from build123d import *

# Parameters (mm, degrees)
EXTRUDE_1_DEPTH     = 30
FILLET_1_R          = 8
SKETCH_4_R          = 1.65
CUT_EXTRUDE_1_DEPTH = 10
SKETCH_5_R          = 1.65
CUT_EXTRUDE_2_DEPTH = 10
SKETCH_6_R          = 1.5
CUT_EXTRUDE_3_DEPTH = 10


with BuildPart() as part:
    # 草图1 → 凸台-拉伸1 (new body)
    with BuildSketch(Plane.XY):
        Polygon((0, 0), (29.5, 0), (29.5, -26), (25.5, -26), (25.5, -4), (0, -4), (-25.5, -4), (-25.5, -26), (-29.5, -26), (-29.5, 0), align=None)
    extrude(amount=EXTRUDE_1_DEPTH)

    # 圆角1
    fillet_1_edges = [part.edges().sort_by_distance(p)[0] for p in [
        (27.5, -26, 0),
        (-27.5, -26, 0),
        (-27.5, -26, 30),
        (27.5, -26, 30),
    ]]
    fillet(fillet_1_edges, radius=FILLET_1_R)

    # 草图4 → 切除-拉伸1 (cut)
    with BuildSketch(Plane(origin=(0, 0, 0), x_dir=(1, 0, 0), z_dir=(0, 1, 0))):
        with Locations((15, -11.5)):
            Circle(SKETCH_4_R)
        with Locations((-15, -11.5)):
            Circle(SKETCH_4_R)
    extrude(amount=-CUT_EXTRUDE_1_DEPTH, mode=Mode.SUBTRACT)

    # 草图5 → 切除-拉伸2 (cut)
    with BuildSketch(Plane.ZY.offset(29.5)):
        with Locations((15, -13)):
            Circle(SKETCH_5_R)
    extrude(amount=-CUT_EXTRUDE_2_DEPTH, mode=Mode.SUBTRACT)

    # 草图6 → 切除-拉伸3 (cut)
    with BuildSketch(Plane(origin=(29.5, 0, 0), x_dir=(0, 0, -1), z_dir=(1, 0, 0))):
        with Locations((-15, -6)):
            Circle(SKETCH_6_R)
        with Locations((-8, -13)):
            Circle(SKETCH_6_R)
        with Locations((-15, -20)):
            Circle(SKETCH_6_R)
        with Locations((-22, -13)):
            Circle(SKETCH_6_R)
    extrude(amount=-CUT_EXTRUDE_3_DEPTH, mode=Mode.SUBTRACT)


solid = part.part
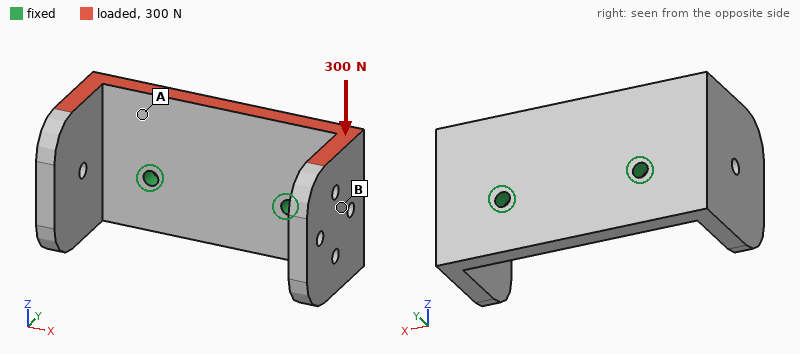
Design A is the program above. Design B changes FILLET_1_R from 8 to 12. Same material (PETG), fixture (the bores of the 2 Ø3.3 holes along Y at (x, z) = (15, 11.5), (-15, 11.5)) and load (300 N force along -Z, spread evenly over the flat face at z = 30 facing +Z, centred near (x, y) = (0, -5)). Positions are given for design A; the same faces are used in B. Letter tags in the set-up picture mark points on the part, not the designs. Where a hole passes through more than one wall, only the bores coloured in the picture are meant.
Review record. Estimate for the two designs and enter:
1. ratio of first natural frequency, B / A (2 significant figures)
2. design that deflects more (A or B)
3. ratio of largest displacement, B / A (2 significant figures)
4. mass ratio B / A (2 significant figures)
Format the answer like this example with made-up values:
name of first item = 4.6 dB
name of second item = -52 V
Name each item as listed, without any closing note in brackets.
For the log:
ratio of first natural frequency, B / A = 1.1
design that deflects more = A
ratio of largest displacement, B / A = 0.60
mass ratio B / A = 0.98
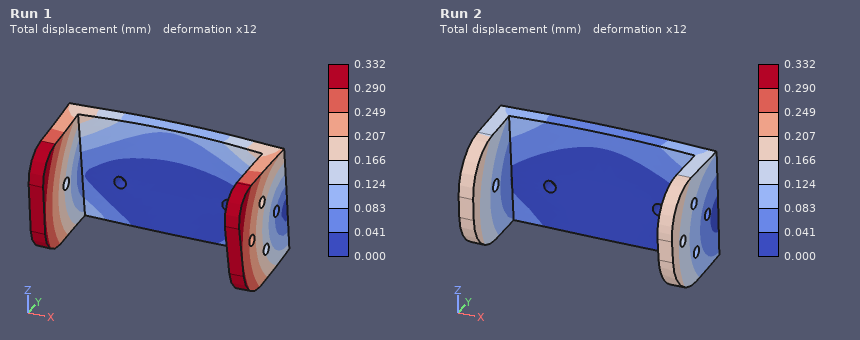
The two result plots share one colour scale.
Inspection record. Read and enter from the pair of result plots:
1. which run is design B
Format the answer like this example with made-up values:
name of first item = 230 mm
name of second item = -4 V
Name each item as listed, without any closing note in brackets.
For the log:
which run is design B = Run 2
